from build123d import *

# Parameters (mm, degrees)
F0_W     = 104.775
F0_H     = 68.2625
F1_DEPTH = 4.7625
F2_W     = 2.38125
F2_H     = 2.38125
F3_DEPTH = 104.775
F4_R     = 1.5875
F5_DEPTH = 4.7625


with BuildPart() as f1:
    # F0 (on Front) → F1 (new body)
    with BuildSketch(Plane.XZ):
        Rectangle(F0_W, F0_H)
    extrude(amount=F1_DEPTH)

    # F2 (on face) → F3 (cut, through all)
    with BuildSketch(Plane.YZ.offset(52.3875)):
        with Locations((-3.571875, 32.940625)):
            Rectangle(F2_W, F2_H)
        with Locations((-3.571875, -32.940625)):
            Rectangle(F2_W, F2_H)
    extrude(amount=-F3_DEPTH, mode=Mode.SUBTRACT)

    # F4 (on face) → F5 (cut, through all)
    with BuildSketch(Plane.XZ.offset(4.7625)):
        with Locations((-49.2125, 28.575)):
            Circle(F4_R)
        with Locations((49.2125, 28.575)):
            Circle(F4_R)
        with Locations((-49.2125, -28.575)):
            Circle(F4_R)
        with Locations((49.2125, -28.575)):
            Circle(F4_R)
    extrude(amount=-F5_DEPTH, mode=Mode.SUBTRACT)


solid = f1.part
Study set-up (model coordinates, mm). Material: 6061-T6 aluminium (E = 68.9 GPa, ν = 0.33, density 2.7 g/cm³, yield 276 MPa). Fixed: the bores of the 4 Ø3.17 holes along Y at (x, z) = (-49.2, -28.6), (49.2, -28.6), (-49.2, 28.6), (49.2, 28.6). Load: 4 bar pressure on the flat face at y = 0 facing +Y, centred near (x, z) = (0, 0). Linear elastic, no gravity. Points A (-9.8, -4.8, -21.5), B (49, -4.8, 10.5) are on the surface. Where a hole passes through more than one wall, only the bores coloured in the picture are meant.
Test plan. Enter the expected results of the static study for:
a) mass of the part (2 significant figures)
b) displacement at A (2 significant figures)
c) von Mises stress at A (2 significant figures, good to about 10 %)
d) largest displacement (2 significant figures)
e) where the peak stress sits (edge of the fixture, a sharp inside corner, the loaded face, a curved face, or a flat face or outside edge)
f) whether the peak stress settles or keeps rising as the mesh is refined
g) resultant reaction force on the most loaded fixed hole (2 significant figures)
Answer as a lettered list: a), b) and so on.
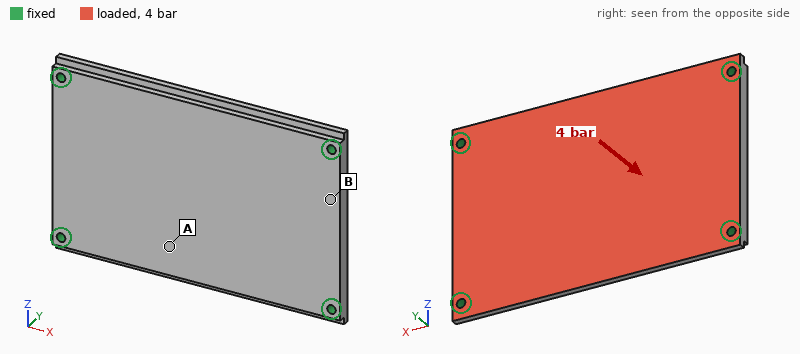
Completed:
a) 88 g
b) 0.26 mm
c) 54 MPa
d) 0.28 mm
e) edge of the fixture
f) keeps rising
g) 710 N
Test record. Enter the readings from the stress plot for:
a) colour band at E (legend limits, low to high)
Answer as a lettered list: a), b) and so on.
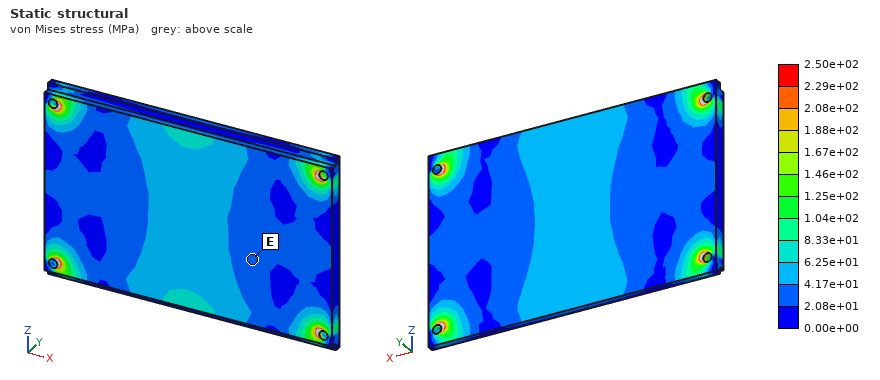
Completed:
a) 2.08e+01 to 4.17e+01 MPa
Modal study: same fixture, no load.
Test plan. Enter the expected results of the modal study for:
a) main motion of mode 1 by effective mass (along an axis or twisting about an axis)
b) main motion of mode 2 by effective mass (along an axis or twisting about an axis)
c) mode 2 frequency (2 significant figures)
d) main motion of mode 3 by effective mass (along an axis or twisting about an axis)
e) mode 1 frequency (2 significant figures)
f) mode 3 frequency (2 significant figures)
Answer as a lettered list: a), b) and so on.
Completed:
a) along Y
b) twisting about X
c) 3300 Hz
d) twisting about Z
e) 1900 Hz
f) 5200 Hz
